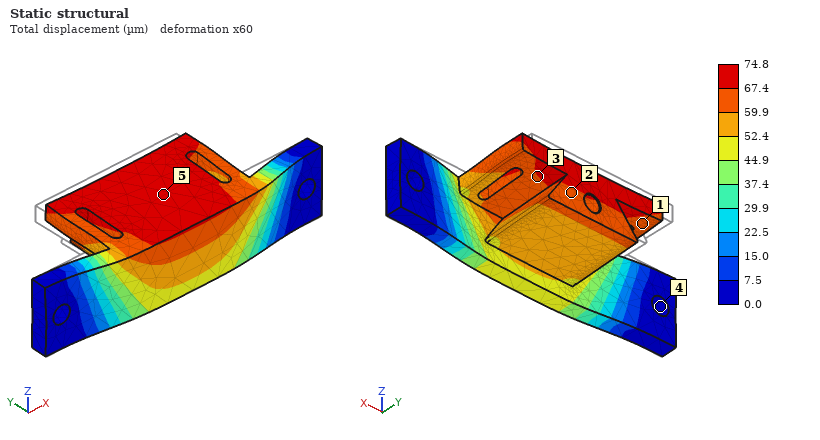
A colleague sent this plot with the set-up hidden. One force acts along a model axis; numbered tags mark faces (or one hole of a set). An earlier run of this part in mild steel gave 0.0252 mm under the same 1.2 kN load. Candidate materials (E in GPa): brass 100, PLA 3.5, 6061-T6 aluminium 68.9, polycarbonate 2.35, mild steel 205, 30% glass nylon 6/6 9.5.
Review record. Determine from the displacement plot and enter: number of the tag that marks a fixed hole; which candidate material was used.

4
6061-T6 aluminium
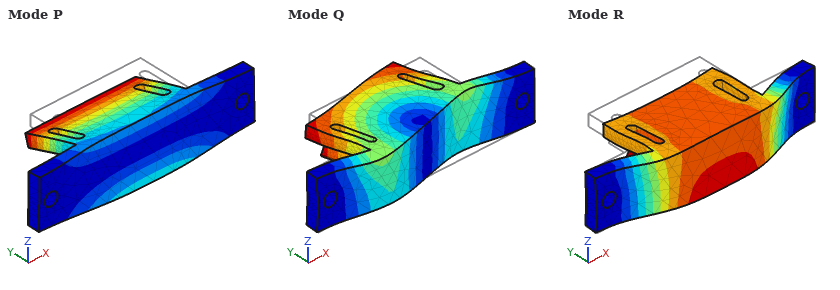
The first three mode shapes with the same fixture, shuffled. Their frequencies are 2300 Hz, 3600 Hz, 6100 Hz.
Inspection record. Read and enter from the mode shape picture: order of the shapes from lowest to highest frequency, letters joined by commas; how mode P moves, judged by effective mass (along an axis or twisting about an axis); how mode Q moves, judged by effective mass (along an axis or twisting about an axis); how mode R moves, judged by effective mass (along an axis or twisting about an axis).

P, R, Q
along Z
along X
along Y
